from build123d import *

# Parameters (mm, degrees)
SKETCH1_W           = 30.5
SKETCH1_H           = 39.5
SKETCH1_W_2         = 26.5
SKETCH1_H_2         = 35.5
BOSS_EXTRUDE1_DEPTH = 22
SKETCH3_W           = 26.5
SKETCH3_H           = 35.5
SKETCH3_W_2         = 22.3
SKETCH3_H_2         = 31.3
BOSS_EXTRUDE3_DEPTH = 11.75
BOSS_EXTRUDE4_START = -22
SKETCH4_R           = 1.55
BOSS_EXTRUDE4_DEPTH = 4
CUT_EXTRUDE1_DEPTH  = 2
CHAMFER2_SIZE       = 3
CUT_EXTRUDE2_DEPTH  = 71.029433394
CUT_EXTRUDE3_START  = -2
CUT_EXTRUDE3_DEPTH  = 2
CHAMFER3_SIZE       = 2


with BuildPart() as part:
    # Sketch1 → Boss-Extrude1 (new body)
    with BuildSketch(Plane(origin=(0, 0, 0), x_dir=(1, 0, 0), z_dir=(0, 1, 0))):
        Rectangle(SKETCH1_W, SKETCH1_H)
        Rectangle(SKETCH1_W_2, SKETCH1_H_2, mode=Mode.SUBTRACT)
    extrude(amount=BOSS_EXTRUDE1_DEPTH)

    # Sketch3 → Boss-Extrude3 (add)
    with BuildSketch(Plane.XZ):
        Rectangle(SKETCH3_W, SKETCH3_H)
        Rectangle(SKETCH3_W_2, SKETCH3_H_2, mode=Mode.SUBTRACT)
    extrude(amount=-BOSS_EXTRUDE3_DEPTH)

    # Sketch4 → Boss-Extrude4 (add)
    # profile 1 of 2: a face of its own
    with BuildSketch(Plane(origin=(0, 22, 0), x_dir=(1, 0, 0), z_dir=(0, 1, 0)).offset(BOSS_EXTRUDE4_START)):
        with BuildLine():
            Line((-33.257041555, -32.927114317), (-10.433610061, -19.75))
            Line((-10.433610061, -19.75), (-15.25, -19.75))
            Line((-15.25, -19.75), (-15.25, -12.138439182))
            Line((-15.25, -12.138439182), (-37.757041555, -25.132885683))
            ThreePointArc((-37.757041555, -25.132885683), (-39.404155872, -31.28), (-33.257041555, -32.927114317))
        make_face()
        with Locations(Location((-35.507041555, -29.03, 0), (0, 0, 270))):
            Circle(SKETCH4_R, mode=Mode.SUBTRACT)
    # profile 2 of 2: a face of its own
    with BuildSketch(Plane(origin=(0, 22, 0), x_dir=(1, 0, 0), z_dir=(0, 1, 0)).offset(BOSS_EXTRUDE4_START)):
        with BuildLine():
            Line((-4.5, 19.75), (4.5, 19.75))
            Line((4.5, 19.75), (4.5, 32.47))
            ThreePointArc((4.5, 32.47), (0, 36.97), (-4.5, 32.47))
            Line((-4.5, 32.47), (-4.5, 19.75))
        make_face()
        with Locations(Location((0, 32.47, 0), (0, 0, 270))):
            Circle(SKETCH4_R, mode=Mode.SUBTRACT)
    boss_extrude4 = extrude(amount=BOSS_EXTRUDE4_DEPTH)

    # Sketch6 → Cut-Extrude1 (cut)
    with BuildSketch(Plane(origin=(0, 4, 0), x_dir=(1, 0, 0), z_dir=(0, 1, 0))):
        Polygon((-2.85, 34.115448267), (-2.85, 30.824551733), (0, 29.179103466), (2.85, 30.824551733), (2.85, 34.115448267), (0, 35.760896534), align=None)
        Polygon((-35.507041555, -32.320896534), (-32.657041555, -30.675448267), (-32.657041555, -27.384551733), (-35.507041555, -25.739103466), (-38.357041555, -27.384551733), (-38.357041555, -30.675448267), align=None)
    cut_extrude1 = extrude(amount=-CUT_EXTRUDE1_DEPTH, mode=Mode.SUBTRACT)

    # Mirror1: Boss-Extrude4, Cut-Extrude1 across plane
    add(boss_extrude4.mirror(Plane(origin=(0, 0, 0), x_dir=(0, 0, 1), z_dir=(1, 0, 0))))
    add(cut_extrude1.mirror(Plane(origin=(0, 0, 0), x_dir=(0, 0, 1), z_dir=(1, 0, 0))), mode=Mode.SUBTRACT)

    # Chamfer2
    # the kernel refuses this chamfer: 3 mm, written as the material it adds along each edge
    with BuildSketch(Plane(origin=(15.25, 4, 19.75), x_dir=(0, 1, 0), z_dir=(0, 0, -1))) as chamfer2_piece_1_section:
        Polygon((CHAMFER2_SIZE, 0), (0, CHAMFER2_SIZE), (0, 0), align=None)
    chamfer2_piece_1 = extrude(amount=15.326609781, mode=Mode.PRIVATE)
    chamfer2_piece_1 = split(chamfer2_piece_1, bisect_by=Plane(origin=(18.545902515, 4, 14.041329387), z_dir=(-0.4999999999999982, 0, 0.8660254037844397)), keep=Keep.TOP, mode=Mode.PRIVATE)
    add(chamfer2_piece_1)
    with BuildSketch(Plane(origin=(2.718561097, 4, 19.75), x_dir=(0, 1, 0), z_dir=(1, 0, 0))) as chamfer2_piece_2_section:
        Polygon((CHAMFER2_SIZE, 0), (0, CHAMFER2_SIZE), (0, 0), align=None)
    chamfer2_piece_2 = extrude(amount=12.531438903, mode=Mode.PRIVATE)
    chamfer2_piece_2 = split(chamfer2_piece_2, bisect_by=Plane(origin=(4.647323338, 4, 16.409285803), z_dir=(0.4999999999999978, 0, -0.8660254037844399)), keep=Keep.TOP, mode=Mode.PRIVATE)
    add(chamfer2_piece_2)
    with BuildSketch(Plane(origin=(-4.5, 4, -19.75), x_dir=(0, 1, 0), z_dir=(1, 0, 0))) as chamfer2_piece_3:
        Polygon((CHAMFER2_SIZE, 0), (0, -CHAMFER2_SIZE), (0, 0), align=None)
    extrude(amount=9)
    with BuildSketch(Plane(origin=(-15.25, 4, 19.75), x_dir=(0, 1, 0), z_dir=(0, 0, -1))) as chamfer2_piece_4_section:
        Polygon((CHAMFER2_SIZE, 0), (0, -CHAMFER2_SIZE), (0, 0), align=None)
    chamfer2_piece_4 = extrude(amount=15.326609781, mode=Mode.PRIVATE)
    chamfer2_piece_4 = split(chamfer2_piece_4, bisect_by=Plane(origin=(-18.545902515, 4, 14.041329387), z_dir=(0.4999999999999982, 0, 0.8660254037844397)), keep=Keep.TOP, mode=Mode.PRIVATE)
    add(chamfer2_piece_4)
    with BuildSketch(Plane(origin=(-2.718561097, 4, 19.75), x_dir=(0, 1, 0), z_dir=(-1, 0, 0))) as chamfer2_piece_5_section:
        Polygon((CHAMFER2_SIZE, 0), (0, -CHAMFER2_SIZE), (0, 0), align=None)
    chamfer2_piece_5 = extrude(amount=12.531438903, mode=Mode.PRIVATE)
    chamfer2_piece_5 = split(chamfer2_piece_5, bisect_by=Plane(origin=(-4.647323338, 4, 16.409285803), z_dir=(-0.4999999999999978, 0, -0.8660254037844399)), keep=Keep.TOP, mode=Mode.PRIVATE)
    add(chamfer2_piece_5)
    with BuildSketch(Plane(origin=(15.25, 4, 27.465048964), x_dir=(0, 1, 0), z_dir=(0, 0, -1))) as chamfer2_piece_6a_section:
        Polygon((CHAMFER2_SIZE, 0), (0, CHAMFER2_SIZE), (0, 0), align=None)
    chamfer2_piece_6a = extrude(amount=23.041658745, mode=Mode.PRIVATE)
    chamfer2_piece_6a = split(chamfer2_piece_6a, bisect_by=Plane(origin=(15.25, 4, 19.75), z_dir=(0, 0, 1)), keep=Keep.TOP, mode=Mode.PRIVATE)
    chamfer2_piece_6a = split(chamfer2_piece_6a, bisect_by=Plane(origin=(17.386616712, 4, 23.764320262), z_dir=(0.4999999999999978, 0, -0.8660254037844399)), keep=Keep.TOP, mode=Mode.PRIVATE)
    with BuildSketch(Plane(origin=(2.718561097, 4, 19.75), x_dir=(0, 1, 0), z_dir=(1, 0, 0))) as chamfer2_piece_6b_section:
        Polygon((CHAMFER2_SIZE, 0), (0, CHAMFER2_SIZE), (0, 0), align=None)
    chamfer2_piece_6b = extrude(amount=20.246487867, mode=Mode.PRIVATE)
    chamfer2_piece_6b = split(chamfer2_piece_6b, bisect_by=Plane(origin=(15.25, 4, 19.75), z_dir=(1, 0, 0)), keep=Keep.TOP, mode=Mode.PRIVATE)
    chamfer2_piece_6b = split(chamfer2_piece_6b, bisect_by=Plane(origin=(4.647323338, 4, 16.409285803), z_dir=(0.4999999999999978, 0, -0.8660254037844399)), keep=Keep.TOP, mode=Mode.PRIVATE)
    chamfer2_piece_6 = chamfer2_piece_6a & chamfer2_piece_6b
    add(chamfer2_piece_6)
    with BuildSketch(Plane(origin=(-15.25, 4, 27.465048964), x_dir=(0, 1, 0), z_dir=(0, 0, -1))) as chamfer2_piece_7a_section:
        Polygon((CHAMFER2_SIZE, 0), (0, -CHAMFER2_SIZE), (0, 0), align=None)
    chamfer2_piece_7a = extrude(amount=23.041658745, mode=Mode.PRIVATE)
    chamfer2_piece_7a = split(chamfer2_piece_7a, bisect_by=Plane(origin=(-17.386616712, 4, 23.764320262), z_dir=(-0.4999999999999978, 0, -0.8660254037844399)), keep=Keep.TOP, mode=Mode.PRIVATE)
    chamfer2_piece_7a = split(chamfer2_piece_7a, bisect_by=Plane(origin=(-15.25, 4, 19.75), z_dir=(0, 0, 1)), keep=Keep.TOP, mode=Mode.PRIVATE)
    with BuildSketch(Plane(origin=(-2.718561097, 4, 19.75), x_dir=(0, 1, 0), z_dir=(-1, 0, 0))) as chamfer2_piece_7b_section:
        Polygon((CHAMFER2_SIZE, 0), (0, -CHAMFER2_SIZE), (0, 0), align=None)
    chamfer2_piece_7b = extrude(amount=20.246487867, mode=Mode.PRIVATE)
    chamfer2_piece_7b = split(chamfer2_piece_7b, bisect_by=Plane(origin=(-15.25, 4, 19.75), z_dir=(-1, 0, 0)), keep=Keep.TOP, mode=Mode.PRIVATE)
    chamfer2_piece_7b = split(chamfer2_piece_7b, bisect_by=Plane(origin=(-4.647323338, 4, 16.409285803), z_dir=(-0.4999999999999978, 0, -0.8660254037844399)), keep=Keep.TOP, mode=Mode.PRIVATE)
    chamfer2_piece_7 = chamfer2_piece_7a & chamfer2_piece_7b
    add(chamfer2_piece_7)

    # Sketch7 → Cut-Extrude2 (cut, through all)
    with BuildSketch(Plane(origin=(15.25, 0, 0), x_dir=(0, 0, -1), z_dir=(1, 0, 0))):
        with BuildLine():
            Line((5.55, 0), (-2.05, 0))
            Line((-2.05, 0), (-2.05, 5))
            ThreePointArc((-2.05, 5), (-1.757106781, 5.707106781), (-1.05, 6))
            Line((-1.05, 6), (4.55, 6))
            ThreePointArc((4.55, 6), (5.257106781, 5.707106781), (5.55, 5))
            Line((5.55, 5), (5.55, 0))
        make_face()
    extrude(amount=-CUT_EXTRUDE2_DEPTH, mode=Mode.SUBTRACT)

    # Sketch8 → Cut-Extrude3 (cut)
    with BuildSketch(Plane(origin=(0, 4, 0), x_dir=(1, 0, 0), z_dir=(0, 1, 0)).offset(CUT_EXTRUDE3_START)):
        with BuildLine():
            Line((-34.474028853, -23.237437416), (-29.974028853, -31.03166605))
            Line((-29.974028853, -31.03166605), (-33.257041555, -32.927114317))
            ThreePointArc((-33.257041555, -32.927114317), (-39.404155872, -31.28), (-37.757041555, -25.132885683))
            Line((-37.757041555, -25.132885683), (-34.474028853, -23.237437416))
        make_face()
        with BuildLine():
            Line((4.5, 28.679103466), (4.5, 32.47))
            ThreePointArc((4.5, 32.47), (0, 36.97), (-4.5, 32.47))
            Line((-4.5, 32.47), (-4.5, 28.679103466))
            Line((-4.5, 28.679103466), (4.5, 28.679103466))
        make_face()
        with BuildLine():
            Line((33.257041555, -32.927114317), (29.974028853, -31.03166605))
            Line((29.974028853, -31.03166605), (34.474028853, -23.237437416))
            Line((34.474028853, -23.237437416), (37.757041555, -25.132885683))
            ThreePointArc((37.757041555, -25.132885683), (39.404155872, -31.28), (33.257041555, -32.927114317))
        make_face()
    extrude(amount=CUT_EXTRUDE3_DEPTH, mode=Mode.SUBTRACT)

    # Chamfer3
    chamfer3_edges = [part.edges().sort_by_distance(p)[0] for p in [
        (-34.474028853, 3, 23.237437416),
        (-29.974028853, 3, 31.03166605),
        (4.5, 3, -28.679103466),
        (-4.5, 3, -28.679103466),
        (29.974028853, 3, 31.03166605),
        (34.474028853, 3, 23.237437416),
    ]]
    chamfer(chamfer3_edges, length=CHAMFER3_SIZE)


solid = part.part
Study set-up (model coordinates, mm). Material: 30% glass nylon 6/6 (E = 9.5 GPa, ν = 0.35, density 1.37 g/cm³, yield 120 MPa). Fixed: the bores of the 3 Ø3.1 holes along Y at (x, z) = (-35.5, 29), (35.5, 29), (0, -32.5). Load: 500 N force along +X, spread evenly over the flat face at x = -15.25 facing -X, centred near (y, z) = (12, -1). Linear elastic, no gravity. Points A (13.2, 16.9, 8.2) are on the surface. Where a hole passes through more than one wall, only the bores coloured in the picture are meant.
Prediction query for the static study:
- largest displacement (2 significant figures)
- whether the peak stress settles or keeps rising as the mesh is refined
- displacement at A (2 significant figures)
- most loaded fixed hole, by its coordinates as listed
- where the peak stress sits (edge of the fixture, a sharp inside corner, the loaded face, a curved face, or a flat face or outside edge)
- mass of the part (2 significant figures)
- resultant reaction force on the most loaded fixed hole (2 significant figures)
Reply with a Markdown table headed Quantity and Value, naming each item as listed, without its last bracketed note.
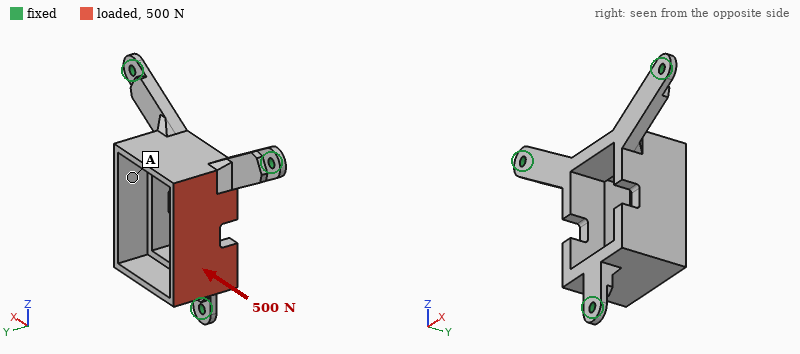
| Quantity | Value |
|---|---|
| largest displacement | 0.94 mm |
| whether the peak stress settles or keeps rising as the mesh is refined | keeps rising |
| displacement at A | 0.27 mm |
| most loaded fixed hole, by its coordinates as listed | (35.5, 29) |
| where the peak stress sits | edge of the fixture |
| mass of the part | 14 g |
| resultant reaction force on the most loaded fixed hole | 260 N |
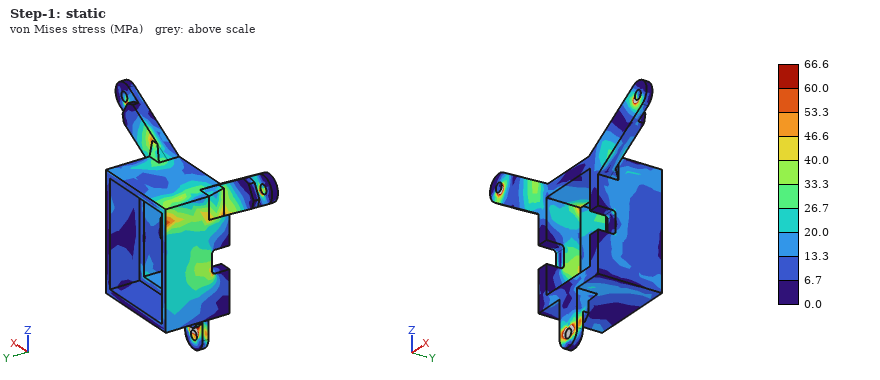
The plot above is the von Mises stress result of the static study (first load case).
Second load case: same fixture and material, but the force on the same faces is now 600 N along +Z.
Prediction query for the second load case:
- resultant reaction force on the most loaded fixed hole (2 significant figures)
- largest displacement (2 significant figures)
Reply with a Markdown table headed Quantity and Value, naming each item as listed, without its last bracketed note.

| Quantity | Value |
|---|---|
| resultant reaction force on the most loaded fixed hole | 350 N |
| largest displacement | 0.40 mm |
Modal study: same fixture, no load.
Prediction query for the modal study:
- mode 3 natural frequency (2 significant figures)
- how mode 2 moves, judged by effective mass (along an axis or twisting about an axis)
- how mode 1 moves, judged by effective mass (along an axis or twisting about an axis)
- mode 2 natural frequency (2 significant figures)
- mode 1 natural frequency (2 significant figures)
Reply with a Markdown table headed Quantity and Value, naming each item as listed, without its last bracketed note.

| Quantity | Value |
|---|---|
| mode 3 natural frequency | 2900 Hz |
| how mode 2 moves, judged by effective mass | along Y |
| how mode 1 moves, judged by effective mass | along X |
| mode 2 natural frequency | 1500 Hz |
| mode 1 natural frequency | 1400 Hz |
